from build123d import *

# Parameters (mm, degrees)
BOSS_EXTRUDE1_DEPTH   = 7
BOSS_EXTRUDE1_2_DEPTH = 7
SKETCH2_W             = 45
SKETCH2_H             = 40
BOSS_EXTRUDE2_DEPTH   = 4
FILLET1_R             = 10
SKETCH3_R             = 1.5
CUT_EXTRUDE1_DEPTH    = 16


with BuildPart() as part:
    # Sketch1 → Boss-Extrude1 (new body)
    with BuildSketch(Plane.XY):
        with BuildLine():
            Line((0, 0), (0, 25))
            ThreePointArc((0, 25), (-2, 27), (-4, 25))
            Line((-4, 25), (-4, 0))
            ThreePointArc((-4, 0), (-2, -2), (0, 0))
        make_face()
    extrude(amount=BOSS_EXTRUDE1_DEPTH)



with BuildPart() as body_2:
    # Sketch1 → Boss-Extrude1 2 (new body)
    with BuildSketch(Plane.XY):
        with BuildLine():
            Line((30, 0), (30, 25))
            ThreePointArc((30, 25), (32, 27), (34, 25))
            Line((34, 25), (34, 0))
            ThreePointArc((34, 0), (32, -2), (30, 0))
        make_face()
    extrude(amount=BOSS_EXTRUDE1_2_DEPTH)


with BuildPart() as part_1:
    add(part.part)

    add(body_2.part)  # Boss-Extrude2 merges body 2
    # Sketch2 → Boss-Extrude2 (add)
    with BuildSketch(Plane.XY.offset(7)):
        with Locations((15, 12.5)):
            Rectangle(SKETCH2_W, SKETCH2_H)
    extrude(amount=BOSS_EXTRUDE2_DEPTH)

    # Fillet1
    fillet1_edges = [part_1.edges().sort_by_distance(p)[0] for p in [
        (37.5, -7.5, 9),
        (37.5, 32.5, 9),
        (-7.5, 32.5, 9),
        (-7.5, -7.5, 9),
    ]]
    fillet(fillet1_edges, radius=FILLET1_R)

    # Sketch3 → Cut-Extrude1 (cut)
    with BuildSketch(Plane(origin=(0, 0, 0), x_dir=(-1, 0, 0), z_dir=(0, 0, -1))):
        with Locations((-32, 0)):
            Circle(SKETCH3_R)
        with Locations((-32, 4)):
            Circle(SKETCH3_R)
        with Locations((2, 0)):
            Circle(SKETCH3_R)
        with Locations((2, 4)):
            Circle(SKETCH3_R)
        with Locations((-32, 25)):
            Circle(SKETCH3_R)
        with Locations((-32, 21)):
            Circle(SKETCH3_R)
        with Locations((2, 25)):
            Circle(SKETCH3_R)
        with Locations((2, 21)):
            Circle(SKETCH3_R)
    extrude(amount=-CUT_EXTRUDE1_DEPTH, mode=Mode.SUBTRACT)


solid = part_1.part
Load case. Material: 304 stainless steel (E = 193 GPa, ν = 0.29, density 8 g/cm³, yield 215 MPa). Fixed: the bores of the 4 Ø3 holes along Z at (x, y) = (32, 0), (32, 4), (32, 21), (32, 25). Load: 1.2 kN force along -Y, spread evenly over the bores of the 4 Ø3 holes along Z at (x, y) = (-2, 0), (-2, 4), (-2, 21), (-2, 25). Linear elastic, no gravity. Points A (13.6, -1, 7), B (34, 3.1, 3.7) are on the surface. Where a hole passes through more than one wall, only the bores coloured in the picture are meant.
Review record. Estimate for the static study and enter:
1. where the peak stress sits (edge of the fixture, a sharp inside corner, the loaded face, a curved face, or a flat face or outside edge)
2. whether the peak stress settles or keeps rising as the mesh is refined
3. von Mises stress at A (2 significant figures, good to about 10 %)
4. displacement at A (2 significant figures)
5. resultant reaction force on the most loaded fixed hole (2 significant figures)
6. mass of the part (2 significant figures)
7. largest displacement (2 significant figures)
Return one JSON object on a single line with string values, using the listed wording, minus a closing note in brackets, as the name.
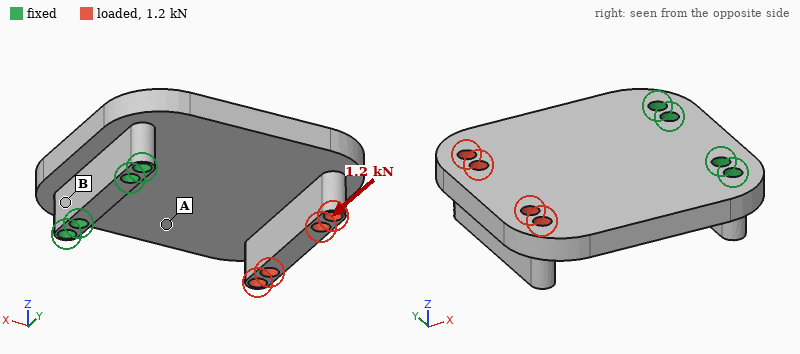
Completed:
{"where the peak stress sits": "edge of the fixture", "whether the peak stress settles or keeps rising as the mesh is refined": "keeps rising", "von Mises stress at A": "36 MPa", "displacement at A": "11 µm", "resultant reaction force on the most loaded fixed hole": "1.3 kN", "mass of the part": "62 g", "largest displacement": "34 µm"}
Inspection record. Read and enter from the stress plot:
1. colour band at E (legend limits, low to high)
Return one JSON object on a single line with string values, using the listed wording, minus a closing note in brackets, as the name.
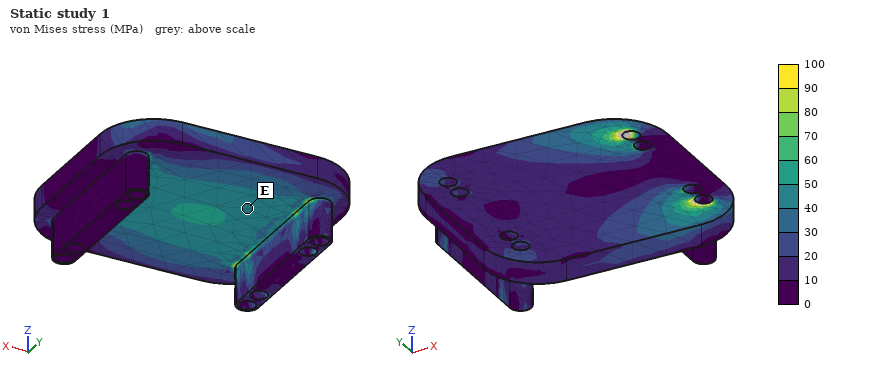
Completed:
{"colour band at E": "40 to 50 MPa"}
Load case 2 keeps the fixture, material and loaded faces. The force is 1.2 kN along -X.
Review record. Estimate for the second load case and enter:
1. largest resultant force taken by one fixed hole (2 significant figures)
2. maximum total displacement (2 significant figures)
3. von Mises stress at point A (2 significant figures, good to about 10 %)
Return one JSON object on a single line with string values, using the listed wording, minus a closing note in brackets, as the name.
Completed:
{"largest resultant force taken by one fixed hole": "320 N", "maximum total displacement": "74 µm", "von Mises stress at point A": "45 MPa"}
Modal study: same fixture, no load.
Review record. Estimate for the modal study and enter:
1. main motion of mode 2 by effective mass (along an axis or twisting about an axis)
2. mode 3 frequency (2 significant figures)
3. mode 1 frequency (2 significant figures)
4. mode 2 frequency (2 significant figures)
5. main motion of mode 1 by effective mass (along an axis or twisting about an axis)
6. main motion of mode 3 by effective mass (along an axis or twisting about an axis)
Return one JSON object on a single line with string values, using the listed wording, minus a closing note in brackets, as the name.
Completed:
{"main motion of mode 2 by effective mass": "twisting about X", "mode 3 frequency": "11 kHz", "mode 1 frequency": "2000 Hz", "mode 2 frequency": "5000 Hz", "main motion of mode 1 by effective mass": "along Z", "main motion of mode 3 by effective mass": "along Y"}
